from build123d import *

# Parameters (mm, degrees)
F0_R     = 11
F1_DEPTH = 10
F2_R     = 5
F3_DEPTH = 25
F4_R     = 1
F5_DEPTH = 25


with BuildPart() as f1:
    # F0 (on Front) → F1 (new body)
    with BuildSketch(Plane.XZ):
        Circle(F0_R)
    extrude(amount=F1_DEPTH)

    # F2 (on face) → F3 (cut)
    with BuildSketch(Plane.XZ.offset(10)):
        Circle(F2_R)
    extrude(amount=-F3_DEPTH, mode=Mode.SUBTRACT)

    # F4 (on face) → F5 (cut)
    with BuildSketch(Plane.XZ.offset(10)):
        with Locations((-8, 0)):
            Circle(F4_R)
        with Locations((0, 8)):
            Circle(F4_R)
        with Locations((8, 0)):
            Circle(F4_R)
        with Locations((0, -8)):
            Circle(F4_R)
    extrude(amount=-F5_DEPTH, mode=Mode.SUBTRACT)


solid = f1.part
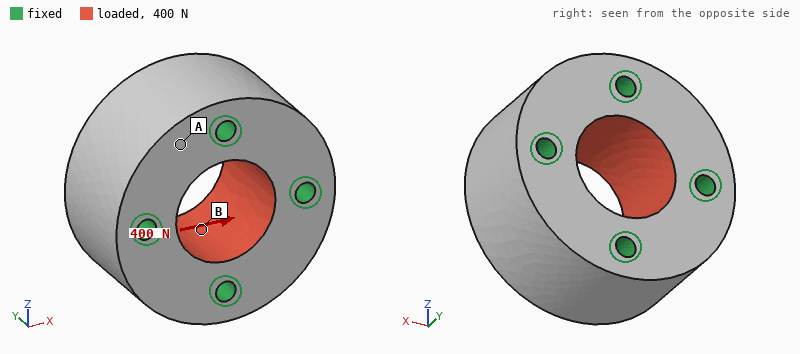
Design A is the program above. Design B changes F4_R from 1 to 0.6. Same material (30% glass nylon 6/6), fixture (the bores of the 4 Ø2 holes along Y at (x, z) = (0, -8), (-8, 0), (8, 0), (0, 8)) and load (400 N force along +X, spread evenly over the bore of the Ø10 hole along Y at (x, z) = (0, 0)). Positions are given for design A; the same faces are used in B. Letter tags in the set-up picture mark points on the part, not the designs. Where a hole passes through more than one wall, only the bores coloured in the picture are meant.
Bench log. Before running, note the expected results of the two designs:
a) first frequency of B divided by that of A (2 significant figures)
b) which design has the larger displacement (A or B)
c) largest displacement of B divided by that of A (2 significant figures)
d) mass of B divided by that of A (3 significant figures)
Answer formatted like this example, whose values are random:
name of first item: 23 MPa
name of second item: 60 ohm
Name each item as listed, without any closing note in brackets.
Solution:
first frequency of B divided by that of A: 0.88
which design has the larger displacement: B
largest displacement of B divided by that of A: 1.2
mass of B divided by that of A: 1.03
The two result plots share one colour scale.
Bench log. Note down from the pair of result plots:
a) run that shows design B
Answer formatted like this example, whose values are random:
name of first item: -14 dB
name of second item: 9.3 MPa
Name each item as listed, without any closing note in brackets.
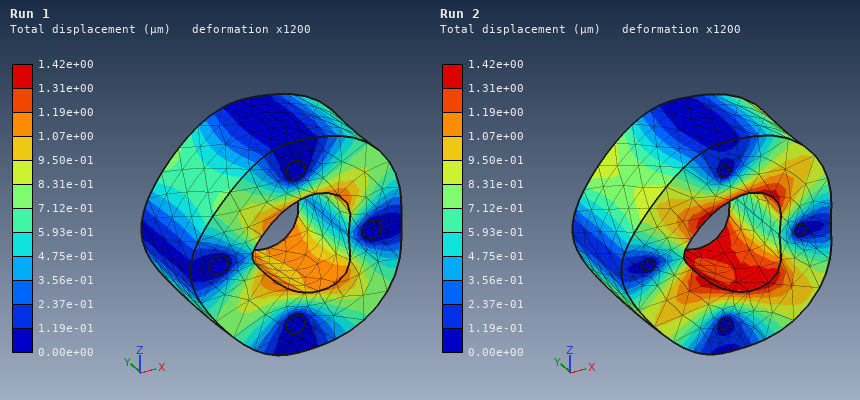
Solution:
run that shows design B: Run 2
